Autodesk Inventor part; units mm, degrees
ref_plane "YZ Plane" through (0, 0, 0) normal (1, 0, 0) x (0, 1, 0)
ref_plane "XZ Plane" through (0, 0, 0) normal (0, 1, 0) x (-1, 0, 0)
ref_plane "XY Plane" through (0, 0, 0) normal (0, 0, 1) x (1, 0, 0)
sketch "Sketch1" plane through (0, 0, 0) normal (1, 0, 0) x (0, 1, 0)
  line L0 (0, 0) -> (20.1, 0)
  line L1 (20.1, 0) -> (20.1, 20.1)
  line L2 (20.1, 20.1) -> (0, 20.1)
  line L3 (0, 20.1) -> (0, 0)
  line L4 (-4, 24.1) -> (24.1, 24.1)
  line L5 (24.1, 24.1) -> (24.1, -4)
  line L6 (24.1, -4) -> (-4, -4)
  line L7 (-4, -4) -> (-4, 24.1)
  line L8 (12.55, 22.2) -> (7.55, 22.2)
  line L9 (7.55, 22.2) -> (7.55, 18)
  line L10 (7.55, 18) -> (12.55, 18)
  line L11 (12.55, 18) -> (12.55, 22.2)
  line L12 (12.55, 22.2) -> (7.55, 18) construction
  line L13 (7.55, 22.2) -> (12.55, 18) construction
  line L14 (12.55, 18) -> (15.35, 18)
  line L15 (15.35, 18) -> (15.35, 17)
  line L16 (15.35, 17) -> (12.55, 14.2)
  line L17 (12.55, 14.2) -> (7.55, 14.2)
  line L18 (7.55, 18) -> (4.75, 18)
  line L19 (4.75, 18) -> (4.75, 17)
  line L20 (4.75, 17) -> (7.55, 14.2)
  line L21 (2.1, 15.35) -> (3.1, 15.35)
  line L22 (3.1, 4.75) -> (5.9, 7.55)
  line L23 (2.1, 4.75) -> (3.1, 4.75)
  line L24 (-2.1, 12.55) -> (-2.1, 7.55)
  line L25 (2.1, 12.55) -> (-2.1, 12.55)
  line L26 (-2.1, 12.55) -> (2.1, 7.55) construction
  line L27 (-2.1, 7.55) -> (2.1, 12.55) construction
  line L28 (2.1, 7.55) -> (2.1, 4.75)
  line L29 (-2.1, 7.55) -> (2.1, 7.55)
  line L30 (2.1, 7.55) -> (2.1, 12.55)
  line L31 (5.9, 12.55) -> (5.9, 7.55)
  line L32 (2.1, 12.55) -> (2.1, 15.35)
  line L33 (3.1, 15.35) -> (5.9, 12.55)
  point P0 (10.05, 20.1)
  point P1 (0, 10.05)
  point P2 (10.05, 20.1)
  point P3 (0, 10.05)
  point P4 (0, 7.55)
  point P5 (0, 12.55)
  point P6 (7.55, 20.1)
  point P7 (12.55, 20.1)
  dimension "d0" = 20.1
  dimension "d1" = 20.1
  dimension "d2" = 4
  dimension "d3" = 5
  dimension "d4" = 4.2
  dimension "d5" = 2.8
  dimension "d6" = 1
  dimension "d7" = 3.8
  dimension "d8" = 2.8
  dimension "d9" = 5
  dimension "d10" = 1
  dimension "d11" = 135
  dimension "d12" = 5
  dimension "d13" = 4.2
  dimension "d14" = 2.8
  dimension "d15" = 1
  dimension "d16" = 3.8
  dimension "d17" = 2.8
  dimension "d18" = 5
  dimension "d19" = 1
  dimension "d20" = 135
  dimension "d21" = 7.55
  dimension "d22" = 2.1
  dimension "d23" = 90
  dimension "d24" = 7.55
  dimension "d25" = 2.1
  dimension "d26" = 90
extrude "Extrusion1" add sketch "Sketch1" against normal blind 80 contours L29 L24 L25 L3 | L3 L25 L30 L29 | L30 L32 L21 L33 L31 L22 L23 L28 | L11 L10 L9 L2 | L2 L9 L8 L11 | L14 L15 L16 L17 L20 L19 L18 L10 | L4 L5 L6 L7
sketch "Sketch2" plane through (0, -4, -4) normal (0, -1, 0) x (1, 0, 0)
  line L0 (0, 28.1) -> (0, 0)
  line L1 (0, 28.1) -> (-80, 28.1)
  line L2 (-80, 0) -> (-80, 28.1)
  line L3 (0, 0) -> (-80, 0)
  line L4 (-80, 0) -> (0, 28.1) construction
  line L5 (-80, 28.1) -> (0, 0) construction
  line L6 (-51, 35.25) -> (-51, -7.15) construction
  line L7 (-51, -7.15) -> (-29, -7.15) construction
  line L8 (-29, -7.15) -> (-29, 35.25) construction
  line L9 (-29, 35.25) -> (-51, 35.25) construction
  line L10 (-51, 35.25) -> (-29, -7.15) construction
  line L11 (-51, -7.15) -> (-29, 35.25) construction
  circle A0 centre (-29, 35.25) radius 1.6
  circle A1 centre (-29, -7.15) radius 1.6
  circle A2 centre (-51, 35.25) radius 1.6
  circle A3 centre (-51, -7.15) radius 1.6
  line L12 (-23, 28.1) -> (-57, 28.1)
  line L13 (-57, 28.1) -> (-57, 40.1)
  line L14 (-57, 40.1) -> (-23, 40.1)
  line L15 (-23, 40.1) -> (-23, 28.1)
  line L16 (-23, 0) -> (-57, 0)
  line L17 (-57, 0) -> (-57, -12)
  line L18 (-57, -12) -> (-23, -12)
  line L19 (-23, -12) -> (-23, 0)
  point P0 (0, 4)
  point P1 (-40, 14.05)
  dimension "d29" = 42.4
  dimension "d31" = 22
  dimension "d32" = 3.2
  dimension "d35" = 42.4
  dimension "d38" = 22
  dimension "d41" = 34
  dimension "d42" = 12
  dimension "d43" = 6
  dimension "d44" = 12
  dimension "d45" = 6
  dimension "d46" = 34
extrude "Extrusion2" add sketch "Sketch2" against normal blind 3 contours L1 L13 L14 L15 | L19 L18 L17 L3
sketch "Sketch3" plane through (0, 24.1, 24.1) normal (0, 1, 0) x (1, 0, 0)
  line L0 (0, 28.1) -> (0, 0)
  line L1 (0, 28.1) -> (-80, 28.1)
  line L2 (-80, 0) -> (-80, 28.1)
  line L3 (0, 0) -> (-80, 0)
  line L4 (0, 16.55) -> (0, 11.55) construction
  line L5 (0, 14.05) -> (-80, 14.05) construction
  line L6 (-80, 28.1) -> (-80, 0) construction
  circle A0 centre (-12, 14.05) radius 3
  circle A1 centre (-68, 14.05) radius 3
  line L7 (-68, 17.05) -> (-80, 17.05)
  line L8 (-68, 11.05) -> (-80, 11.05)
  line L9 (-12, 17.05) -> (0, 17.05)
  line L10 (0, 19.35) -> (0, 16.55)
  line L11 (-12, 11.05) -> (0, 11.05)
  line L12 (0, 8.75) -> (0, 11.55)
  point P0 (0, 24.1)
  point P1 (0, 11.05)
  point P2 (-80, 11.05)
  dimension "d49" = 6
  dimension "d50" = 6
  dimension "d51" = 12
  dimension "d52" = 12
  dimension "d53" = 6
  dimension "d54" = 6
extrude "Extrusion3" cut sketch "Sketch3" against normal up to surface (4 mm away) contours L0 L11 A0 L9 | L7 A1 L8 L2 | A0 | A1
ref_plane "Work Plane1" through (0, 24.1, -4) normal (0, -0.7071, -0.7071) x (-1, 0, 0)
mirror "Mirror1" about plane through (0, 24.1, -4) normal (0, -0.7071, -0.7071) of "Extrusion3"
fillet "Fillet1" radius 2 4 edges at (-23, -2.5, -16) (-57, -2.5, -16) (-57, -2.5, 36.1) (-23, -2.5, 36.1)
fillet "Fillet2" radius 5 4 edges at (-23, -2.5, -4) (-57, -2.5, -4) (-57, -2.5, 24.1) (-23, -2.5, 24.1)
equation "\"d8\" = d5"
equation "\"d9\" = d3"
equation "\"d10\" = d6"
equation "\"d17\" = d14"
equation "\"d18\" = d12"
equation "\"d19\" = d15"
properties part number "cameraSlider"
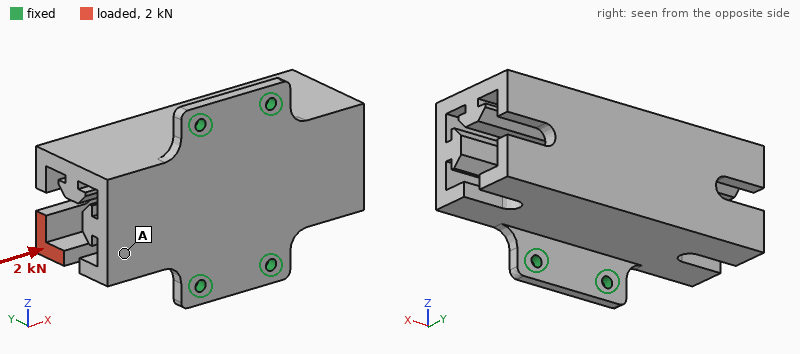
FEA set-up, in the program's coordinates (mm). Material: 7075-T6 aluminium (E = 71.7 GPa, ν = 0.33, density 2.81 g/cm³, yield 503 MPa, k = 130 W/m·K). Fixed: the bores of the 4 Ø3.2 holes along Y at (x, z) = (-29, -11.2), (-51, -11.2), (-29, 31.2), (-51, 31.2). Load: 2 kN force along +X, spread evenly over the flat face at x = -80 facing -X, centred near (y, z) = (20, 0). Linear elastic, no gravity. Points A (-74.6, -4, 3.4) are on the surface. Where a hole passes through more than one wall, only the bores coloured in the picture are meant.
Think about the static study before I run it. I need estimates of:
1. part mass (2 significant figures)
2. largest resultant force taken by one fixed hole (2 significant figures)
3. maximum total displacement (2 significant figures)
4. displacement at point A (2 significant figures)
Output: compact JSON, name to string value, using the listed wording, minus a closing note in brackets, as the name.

{"part mass": "110 g", "largest resultant force taken by one fixed hole": "1.2 kN", "maximum total displacement": "0.17 mm", "displacement at point A": "0.11 mm"}
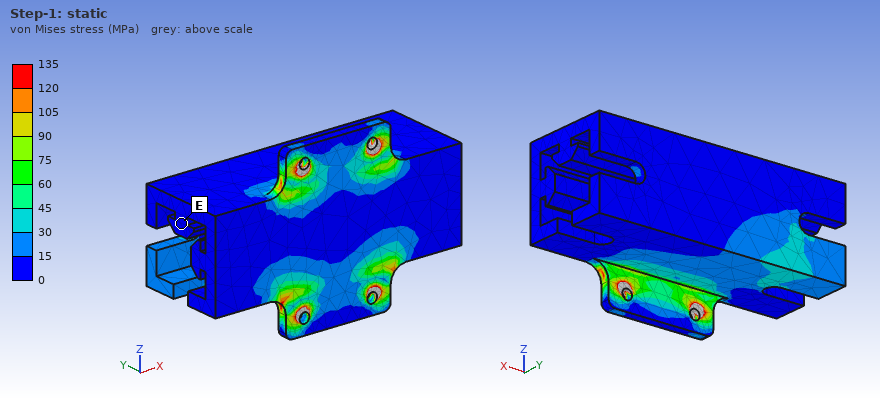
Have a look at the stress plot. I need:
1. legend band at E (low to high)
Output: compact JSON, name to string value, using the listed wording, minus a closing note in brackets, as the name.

{"legend band at E": "0 to 15 MPa"}
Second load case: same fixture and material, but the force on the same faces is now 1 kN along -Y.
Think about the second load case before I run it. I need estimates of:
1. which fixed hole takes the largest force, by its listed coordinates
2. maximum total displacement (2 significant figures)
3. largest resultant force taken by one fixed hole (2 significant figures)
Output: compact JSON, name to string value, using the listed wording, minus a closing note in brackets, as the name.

{"which fixed hole takes the largest force, by its listed coordinates": "(-51, -11.2)", "maximum total displacement": "0.25 mm", "largest resultant force taken by one fixed hole": "1.3 kN"}
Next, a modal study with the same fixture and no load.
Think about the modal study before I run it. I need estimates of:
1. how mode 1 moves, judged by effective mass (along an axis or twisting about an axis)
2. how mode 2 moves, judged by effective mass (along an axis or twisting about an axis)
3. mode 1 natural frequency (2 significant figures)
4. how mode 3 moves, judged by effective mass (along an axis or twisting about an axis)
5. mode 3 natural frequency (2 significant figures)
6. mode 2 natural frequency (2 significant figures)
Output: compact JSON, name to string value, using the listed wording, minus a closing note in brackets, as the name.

{"how mode 1 moves, judged by effective mass": "along X", "how mode 2 moves, judged by effective mass": "along Z", "mode 1 natural frequency": "2200 Hz", "how mode 3 moves, judged by effective mass": "along Y", "mode 3 natural frequency": "4800 Hz", "mode 2 natural frequency": "3900 Hz"}
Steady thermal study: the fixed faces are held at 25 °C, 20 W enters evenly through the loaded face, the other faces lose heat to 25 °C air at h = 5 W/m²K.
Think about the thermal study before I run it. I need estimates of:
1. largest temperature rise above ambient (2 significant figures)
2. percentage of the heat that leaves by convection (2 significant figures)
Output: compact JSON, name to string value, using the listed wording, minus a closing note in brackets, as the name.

{"largest temperature rise above ambient": "63 K", "percentage of the heat that leaves by convection": "5.6 %"}
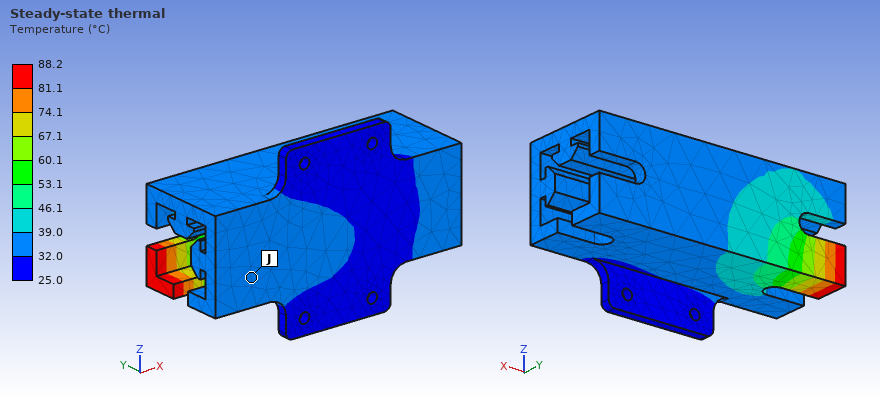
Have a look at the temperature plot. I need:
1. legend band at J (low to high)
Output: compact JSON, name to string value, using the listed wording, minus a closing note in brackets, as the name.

{"legend band at J": "32.0 to 39.0 °C"}
